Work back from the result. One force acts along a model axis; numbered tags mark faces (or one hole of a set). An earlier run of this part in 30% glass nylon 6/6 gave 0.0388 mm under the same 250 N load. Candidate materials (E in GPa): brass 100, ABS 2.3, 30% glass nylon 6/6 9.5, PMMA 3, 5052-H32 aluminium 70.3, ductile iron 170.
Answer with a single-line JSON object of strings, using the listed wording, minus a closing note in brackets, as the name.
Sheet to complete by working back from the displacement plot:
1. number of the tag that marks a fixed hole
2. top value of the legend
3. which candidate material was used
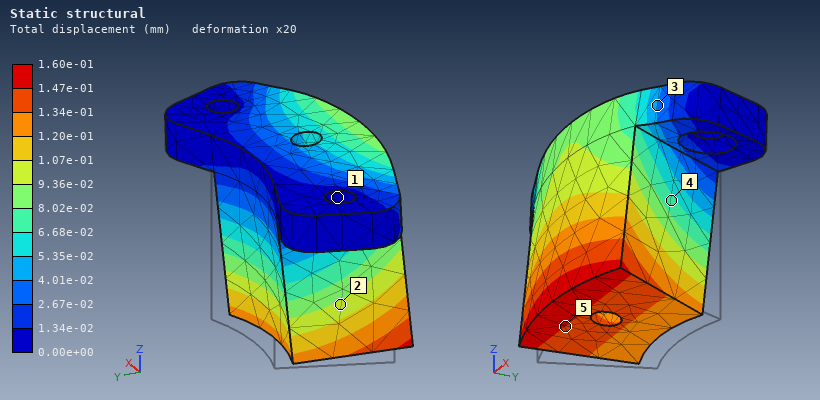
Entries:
{"number of the tag that marks a fixed hole": "1", "top value of the legend": "1.60e-01 mm", "which candidate material was used": "ABS"}
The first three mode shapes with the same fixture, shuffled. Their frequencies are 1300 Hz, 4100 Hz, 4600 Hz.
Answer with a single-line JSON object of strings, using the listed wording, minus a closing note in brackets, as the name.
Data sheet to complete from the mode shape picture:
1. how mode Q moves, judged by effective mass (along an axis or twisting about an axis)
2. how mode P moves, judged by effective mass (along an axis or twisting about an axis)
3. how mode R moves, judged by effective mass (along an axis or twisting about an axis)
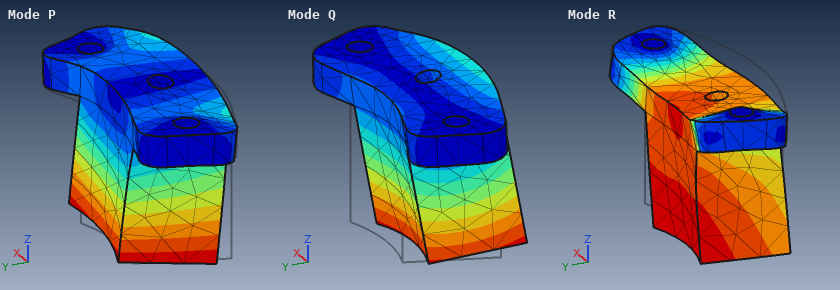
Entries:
{"how mode Q moves, judged by effective mass": "along Y", "how mode P moves, judged by effective mass": "along X", "how mode R moves, judged by effective mass": "along Z"}
